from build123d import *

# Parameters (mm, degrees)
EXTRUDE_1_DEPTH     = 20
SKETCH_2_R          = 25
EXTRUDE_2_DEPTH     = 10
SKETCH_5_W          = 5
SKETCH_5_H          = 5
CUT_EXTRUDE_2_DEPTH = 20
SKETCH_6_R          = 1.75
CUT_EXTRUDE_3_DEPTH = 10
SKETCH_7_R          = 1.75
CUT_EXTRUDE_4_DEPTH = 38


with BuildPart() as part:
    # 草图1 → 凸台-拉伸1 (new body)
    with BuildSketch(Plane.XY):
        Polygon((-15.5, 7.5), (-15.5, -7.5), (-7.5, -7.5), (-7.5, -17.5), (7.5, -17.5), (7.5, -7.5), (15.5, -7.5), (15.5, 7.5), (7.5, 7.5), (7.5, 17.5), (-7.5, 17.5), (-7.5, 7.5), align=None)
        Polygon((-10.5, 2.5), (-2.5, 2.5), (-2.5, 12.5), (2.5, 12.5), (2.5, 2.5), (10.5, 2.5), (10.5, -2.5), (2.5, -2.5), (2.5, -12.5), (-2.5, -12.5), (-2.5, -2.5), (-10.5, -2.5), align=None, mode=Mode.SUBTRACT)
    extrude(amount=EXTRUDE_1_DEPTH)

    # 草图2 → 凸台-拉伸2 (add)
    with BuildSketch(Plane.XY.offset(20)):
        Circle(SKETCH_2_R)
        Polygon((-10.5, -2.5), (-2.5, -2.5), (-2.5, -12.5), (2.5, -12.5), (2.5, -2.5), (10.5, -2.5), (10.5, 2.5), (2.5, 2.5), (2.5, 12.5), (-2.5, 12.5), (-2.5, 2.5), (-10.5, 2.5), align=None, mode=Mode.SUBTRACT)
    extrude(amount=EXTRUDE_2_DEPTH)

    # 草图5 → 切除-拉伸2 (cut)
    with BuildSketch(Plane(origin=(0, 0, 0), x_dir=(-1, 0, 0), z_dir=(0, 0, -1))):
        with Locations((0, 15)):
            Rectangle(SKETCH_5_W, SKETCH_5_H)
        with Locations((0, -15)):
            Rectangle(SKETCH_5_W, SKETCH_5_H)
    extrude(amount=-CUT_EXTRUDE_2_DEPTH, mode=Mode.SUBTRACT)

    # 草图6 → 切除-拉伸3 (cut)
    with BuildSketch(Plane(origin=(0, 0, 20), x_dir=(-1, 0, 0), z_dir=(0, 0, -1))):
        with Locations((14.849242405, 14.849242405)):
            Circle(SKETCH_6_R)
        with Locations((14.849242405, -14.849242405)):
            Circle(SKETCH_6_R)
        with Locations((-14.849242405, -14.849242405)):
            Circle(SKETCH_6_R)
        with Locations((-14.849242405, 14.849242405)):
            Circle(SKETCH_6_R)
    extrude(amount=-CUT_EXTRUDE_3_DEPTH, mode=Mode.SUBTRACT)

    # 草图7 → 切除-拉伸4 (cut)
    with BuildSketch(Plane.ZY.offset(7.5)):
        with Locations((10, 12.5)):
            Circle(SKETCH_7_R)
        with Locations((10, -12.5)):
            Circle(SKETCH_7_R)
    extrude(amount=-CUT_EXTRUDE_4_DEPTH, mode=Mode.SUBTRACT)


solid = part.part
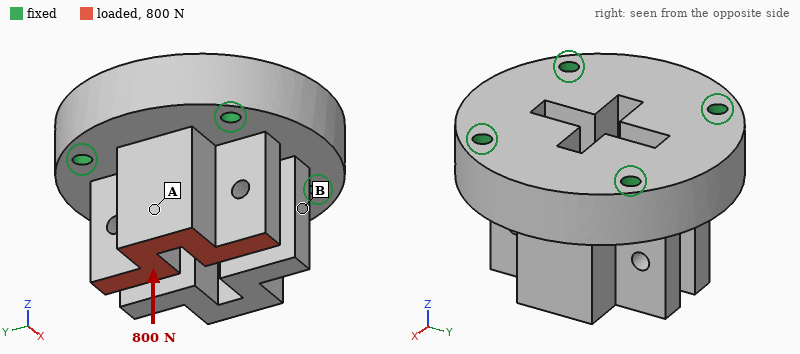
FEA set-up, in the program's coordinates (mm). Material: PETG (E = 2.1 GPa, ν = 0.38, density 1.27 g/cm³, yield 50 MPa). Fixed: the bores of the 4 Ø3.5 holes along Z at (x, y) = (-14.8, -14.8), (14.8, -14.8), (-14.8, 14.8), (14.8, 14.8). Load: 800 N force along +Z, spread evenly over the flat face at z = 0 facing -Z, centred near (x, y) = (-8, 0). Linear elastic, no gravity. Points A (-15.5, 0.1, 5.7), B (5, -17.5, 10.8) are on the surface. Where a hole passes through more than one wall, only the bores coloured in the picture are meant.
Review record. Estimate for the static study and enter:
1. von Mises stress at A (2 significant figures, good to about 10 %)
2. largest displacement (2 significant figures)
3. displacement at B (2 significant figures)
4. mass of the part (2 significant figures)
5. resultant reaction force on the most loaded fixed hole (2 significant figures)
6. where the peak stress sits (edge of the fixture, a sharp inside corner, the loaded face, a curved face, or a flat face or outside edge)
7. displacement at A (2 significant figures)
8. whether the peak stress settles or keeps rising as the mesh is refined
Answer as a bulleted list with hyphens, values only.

- 4.0 MPa
- 0.12 mm
- 0.025 mm
- 35 g
- 330 N
- edge of the fixture
- 0.065 mm
- keeps rising
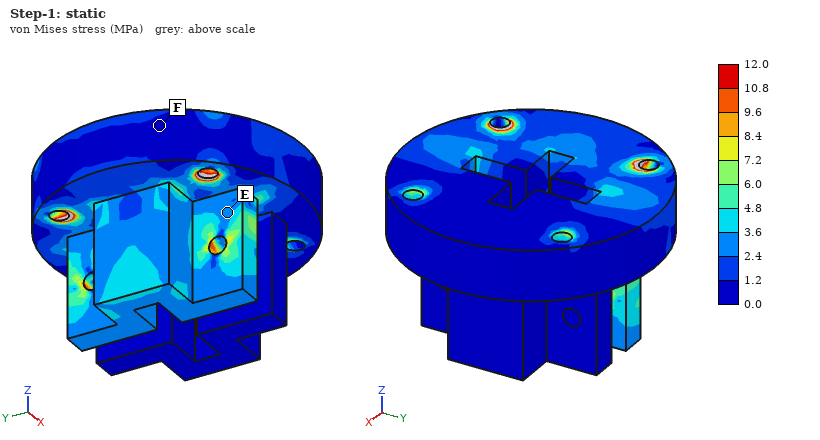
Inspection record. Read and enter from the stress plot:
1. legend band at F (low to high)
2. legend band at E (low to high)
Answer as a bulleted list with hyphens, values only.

- 0.0 to 1.2 MPa
- 2.4 to 3.6 MPa
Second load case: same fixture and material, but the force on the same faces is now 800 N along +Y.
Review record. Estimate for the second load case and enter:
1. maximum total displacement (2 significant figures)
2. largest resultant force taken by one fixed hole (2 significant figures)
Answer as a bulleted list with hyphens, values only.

- 0.54 mm
- 570 N
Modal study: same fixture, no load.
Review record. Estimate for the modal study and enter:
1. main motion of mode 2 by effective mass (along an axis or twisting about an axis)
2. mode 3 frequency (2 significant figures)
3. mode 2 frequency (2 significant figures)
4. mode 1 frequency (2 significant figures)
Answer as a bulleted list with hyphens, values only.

- along X
- 3500 Hz
- 2900 Hz
- 2600 Hz
